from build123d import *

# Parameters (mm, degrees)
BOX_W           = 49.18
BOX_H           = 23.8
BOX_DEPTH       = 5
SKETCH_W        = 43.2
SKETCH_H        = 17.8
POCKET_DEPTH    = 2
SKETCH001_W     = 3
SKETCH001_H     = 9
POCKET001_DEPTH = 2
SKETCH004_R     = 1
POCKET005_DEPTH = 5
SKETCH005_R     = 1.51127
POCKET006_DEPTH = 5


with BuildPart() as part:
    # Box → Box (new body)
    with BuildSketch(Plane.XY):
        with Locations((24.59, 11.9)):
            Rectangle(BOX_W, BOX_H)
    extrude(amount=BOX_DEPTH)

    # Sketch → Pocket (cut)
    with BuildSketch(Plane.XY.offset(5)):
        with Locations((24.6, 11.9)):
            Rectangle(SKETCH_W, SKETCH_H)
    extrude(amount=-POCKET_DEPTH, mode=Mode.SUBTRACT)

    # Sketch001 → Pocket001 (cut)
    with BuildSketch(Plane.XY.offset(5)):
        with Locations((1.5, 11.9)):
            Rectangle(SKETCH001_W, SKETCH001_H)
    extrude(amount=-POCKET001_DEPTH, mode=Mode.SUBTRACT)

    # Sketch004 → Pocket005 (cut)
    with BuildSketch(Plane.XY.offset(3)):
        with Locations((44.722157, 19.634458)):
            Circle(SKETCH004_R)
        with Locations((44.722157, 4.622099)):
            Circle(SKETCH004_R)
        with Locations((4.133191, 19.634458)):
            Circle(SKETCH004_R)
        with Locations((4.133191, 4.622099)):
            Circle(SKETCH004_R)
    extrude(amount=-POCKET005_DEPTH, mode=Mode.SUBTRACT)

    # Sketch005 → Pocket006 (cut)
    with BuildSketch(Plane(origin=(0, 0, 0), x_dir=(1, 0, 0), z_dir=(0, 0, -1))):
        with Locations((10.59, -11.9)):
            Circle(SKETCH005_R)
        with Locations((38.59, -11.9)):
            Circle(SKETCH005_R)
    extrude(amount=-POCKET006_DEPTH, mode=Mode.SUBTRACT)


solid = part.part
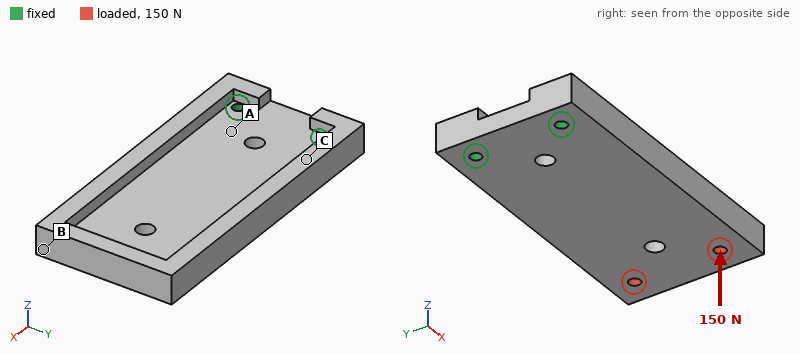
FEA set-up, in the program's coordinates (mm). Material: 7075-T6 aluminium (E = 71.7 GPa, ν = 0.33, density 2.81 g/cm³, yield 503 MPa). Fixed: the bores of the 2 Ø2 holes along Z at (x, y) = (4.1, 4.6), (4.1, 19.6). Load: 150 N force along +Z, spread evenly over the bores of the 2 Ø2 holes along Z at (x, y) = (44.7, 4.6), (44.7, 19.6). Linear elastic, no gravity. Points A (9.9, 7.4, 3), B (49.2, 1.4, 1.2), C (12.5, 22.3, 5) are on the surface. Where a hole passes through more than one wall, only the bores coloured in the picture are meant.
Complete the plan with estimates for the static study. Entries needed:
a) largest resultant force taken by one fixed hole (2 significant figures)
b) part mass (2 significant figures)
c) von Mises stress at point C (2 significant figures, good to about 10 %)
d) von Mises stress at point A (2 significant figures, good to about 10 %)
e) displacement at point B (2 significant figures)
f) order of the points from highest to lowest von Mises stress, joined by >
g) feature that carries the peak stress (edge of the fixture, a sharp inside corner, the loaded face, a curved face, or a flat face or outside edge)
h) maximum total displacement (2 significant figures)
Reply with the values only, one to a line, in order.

110 N
12 g
130 MPa
66 MPa
0.55 mm
C > A > B
edge of the fixture
0.56 mm
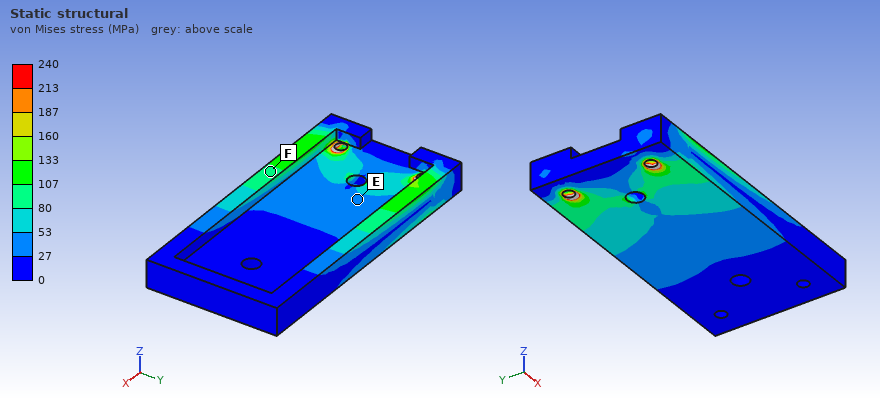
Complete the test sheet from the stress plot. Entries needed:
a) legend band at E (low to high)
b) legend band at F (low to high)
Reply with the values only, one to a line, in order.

27 to 53 MPa
80 to 107 MPa
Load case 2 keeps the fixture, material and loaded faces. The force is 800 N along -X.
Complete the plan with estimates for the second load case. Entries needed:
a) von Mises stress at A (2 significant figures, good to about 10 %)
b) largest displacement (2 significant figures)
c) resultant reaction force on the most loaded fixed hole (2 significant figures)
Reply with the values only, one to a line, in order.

9.0 MPa
34 µm
400 N
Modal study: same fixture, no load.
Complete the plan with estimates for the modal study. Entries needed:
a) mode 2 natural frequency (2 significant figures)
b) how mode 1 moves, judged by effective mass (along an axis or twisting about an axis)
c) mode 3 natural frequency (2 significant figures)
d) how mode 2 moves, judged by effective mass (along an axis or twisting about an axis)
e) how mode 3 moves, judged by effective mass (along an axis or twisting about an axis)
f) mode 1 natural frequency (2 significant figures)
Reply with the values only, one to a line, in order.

4500 Hz
along Z
7100 Hz
twisting about X
along Y
1400 Hz
